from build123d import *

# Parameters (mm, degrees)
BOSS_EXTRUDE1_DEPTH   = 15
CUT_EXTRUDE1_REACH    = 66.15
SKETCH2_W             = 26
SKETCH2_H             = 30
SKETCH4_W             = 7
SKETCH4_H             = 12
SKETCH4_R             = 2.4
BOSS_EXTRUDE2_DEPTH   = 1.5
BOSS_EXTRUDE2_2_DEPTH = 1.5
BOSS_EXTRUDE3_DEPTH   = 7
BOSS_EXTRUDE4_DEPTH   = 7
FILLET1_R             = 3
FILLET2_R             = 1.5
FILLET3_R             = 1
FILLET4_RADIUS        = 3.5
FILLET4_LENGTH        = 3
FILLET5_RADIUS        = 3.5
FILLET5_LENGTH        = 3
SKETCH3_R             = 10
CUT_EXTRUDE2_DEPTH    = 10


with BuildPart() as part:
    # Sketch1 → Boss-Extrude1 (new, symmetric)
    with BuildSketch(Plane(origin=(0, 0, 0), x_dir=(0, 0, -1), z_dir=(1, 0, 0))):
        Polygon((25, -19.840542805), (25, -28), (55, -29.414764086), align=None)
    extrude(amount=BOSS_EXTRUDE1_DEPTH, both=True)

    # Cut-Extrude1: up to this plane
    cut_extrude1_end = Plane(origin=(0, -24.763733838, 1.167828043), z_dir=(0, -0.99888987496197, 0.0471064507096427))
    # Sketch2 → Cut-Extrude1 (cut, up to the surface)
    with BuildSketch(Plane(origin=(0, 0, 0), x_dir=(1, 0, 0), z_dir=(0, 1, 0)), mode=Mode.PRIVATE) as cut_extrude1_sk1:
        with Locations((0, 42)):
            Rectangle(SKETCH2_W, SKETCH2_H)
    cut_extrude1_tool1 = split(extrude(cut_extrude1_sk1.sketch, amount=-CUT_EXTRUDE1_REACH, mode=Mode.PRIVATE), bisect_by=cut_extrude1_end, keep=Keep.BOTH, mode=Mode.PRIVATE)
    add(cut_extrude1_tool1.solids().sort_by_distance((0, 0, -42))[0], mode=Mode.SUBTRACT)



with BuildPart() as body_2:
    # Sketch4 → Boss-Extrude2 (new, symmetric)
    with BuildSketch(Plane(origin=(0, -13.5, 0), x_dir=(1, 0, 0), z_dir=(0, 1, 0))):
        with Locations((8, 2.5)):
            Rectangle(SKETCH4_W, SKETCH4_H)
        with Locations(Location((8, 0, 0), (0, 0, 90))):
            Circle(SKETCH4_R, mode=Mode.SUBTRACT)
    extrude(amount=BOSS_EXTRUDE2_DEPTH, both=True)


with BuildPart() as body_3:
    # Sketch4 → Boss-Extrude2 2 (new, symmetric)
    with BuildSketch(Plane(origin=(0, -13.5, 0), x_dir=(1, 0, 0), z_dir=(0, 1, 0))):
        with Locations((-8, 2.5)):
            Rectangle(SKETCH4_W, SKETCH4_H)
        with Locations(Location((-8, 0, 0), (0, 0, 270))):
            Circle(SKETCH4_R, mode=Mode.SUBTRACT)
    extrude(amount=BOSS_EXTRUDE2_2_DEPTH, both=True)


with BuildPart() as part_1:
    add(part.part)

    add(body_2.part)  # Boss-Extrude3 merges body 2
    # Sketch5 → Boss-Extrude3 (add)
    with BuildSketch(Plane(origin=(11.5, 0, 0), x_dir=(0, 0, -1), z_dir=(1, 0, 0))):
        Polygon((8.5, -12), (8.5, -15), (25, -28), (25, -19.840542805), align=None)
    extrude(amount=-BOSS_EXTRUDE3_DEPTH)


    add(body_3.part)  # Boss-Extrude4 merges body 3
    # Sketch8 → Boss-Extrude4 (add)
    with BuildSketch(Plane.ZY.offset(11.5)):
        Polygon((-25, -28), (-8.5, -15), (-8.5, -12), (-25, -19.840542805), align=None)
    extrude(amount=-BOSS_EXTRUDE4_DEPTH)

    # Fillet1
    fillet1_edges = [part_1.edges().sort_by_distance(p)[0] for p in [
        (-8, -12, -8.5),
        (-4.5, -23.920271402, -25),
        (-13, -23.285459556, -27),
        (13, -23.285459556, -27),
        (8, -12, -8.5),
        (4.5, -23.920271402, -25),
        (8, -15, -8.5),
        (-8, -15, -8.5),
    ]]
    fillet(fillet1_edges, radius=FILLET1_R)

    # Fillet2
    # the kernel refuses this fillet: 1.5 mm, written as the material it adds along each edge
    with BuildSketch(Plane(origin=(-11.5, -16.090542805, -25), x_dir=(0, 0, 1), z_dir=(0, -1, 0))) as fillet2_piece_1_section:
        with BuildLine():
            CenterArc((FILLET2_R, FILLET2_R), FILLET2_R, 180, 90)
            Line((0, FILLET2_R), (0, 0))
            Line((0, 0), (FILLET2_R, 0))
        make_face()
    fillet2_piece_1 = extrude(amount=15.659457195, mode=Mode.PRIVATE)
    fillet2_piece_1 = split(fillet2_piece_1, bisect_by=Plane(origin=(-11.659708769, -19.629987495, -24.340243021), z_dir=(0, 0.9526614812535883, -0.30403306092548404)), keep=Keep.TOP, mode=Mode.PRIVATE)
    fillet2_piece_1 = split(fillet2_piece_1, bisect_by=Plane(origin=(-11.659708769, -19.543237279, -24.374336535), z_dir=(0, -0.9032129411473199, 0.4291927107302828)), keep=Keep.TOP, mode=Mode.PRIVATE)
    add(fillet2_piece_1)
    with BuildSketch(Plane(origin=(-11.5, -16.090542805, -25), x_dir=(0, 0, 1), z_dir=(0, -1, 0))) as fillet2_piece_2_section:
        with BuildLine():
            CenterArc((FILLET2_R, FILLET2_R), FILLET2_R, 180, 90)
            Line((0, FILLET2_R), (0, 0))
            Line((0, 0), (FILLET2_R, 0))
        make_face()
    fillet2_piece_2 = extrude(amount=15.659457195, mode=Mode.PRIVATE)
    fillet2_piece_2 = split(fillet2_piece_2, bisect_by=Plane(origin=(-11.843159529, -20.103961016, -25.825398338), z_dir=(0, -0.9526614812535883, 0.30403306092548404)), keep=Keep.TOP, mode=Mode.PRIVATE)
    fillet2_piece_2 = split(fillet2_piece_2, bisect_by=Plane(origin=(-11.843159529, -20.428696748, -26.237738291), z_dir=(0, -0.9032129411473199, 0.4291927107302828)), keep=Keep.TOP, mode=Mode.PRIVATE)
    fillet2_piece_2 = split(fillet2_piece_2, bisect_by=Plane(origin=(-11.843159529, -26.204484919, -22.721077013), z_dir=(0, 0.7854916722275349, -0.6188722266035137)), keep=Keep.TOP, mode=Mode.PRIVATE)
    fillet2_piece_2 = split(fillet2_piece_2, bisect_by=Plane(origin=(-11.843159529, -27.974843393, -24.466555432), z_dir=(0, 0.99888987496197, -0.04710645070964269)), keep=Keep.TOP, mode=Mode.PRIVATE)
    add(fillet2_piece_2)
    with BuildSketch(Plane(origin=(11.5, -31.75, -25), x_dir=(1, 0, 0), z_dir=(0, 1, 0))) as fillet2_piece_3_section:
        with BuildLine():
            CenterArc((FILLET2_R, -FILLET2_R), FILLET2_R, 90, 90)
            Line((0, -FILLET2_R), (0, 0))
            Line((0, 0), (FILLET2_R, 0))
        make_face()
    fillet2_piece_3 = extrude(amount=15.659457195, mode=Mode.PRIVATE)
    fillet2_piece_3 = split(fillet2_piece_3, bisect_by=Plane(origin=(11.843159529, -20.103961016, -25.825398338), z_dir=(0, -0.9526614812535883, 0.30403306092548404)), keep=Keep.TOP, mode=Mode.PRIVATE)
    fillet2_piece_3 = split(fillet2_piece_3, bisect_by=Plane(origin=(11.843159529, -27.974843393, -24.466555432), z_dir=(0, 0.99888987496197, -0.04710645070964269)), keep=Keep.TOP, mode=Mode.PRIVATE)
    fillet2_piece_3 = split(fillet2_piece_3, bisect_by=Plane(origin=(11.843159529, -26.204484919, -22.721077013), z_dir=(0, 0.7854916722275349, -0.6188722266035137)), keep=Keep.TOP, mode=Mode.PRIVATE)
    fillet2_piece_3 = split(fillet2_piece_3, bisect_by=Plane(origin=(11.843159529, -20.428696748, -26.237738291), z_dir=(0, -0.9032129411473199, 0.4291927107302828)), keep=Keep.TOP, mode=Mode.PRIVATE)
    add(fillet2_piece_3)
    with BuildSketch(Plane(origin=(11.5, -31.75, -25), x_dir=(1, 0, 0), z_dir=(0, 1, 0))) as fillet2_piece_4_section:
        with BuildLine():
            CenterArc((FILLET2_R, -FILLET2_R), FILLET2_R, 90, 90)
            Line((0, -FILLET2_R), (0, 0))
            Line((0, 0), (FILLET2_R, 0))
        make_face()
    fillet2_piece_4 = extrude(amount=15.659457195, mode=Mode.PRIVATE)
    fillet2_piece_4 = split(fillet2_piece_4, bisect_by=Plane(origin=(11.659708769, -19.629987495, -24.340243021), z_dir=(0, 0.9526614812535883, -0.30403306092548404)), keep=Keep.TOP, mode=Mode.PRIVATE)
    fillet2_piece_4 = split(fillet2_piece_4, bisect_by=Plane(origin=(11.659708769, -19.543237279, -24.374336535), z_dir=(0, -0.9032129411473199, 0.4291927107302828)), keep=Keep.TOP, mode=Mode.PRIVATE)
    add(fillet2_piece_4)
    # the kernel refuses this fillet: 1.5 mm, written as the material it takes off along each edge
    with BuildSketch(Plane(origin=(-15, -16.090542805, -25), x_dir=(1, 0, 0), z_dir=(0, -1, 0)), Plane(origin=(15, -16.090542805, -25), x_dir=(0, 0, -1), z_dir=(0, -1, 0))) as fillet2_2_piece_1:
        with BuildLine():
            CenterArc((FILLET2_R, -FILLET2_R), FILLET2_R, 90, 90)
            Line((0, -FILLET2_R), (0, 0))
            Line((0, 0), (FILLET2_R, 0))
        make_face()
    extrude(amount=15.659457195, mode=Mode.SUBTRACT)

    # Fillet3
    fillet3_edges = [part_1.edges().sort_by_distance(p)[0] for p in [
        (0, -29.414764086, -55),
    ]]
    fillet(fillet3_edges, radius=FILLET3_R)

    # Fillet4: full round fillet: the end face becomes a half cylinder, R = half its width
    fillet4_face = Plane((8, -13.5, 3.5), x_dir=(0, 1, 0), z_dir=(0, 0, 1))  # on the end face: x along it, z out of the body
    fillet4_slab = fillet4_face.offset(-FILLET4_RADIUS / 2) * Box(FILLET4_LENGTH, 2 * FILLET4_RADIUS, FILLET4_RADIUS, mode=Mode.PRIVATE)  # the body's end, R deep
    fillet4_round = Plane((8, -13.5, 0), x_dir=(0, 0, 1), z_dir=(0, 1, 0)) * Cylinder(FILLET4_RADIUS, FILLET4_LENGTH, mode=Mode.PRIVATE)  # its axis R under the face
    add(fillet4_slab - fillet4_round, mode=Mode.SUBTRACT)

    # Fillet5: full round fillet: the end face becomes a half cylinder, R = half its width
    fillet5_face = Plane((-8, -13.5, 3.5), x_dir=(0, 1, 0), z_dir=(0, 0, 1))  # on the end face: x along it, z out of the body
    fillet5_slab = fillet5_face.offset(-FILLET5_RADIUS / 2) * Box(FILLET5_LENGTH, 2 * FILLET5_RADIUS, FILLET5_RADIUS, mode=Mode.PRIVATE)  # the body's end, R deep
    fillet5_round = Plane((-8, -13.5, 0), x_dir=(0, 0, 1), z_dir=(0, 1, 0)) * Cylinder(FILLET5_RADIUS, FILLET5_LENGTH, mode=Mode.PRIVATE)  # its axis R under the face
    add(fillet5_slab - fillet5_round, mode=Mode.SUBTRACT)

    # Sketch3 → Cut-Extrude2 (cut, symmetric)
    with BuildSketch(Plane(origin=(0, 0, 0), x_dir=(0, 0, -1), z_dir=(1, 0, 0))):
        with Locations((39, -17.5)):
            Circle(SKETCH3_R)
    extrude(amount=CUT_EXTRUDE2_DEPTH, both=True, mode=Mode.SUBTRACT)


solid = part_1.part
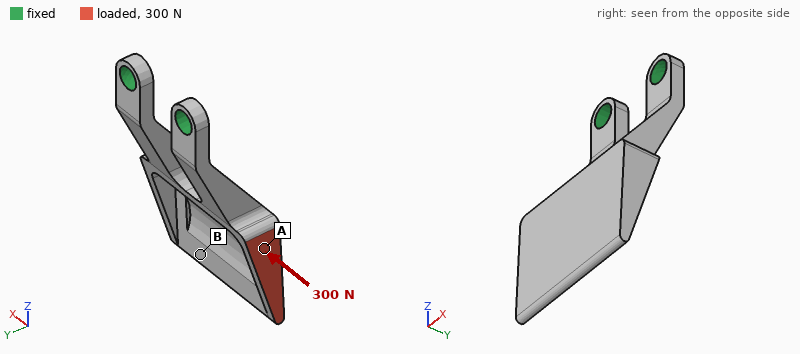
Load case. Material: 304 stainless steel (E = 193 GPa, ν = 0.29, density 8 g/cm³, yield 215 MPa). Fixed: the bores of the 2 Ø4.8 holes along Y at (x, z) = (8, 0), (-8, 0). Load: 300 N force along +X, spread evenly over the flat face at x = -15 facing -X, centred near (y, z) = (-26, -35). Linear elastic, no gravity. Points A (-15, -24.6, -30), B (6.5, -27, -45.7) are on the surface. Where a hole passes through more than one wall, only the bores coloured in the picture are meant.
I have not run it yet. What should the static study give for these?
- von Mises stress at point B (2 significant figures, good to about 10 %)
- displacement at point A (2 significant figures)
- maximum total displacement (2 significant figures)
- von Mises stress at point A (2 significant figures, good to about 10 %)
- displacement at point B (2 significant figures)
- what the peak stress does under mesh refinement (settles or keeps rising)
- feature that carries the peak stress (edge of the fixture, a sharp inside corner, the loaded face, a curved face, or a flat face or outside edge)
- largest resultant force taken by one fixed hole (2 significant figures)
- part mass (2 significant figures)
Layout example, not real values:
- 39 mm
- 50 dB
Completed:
- 9.8 MPa
- 35 µm
- 53 µm
- 26 MPa
- 47 µm
- keeps rising
- edge of the fixture
- 440 N
- 29 g
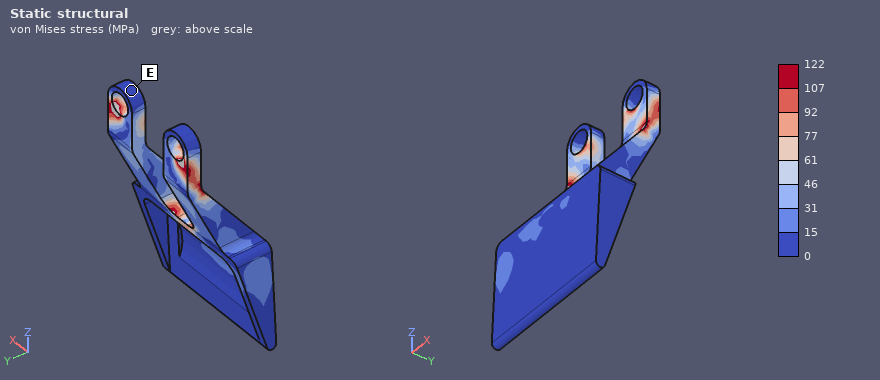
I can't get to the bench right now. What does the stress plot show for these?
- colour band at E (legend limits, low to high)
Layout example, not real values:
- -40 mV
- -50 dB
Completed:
- 0 to 15 MPa
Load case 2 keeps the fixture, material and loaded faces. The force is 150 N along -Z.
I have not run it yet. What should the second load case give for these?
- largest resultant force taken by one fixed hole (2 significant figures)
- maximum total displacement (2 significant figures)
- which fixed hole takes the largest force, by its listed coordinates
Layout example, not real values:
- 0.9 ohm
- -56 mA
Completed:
- 170 N
- 0.19 mm
- (-8, 0)
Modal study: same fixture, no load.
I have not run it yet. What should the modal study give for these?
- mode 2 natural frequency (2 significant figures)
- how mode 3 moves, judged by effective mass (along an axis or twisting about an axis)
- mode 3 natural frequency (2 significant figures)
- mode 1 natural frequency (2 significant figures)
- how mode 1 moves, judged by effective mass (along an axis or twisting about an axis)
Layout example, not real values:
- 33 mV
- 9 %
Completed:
- 2800 Hz
- along X
- 3500 Hz
- 870 Hz
- along Y
